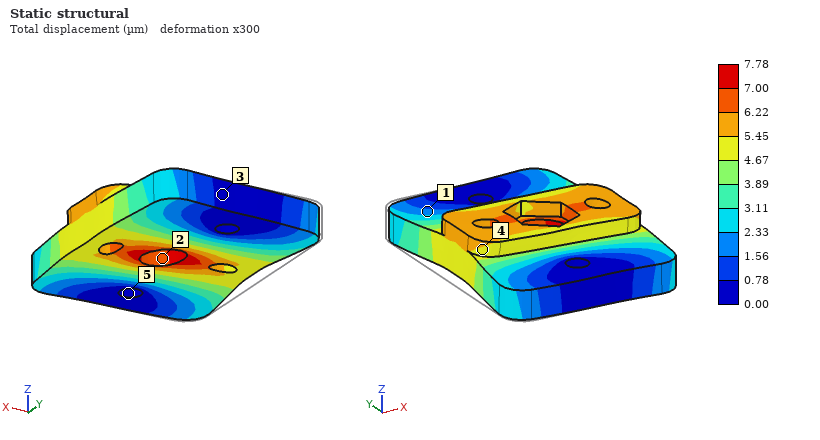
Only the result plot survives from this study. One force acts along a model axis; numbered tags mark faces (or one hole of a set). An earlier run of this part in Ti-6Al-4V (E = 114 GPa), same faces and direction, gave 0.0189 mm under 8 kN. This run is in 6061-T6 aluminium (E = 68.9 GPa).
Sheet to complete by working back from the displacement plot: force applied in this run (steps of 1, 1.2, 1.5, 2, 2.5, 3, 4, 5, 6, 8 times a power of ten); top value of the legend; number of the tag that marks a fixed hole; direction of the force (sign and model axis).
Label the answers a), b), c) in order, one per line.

a) 2 kN
b) 7.78 µm
c) 5
d) +X
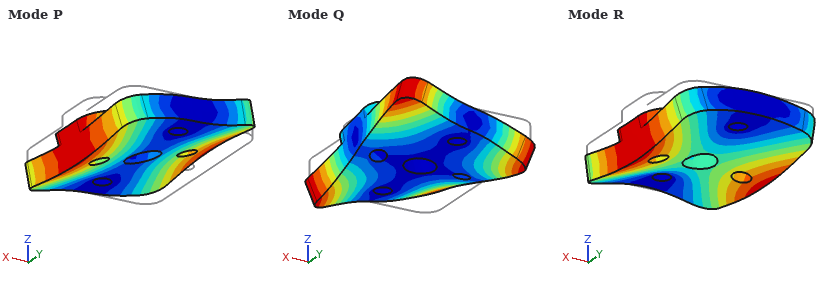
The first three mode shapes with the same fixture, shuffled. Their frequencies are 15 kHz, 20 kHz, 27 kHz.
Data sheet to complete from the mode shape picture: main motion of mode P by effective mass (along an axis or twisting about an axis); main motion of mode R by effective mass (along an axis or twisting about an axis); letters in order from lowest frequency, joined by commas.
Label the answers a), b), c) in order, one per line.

a) twisting about Y
b) along Z
c) P, R, Q
